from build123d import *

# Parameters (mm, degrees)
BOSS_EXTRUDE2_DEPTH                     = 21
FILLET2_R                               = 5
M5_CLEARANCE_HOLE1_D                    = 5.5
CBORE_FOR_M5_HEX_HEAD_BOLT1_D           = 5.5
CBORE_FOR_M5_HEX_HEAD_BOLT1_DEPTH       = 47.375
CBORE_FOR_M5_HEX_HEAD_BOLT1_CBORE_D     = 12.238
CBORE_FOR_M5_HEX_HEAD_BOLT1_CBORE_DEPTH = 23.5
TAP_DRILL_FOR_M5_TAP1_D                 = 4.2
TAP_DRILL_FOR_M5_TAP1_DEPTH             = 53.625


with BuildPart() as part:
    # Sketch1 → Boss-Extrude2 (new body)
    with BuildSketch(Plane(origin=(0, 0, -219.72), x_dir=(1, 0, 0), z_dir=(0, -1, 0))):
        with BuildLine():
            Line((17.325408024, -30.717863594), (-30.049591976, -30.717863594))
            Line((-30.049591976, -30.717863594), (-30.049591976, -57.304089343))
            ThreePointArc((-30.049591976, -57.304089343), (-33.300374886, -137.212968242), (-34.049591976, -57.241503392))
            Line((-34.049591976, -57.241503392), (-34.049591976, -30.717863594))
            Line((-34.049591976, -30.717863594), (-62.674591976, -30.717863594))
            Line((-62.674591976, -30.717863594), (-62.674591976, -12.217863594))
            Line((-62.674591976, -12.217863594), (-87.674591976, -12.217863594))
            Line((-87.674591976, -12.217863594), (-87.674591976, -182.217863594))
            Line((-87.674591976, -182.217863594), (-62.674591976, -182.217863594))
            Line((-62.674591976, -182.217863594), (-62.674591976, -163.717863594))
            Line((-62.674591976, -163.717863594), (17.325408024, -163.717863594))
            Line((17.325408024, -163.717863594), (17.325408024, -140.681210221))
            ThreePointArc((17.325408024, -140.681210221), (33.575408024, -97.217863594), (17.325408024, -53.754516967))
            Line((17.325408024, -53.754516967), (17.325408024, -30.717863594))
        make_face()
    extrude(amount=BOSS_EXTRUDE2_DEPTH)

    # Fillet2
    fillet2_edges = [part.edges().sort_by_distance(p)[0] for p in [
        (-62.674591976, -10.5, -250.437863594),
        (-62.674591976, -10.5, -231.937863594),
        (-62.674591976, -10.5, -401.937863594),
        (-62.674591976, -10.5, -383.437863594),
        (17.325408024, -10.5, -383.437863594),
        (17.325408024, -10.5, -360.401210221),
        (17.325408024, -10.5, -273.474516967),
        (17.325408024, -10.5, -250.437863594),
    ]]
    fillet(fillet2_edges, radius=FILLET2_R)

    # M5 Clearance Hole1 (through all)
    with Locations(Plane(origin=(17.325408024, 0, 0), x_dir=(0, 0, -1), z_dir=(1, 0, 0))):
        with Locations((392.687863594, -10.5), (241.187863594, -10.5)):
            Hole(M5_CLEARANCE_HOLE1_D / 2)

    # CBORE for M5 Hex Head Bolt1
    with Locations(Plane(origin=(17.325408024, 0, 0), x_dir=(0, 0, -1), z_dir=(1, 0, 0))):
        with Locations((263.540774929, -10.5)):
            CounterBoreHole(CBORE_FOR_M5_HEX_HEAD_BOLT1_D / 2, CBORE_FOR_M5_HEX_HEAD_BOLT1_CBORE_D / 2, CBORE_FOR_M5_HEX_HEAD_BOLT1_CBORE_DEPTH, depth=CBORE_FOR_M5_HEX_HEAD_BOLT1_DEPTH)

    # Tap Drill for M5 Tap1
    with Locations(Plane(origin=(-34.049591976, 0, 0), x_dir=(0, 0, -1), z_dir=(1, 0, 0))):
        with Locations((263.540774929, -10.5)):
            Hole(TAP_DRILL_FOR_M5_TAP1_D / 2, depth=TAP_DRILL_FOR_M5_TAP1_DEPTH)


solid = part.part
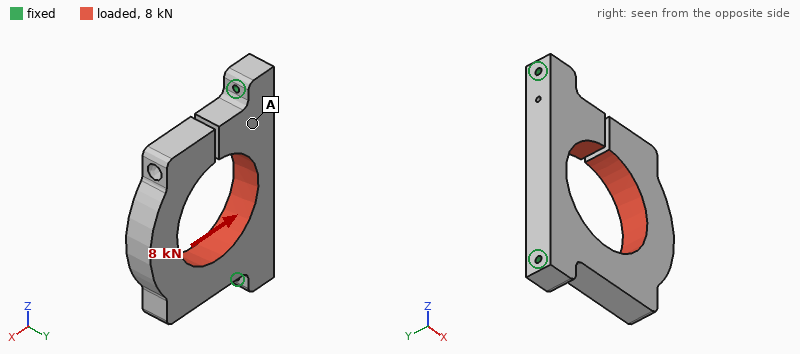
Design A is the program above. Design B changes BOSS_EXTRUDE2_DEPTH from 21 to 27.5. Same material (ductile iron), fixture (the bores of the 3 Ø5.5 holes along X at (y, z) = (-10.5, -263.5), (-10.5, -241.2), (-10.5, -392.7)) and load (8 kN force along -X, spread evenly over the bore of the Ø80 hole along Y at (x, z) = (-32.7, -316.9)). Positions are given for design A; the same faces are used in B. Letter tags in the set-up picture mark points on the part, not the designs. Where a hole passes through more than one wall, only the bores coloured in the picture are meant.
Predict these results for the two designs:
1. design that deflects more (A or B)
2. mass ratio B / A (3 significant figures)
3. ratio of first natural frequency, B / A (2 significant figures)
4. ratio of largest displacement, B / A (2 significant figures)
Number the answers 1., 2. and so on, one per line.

1. A
2. 1.32
3. 1.1
4. 0.87
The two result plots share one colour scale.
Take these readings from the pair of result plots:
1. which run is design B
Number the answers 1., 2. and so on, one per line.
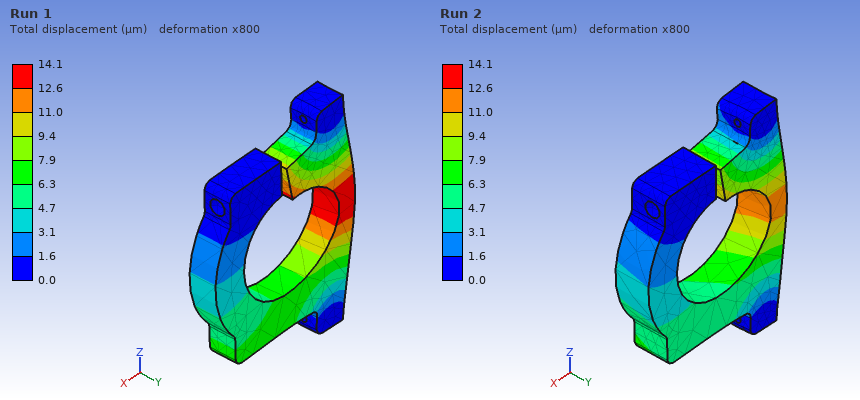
1. Run 2
